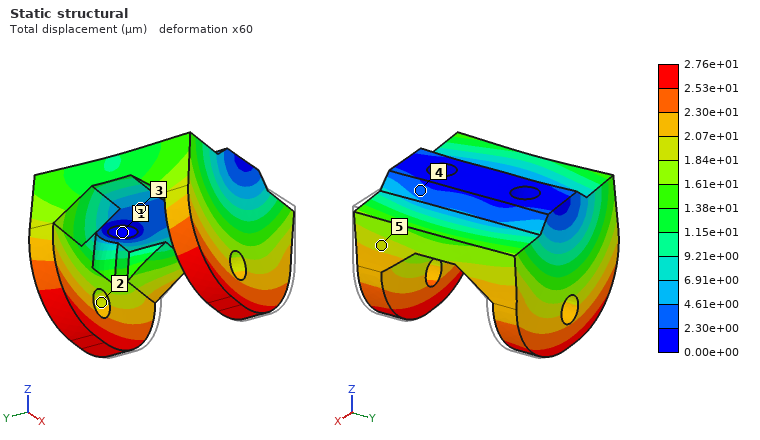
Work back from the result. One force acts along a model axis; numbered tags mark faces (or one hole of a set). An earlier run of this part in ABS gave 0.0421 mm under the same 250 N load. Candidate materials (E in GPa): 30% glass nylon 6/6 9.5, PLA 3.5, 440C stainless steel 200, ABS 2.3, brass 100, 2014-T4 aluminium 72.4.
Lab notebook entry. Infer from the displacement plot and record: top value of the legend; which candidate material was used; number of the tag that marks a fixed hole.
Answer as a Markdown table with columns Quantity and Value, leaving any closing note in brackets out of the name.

| Quantity | Value |
|---|---|
| top value of the legend | 2.76e+01 µm |
| which candidate material was used | PLA |
| number of the tag that marks a fixed hole | 1 |
